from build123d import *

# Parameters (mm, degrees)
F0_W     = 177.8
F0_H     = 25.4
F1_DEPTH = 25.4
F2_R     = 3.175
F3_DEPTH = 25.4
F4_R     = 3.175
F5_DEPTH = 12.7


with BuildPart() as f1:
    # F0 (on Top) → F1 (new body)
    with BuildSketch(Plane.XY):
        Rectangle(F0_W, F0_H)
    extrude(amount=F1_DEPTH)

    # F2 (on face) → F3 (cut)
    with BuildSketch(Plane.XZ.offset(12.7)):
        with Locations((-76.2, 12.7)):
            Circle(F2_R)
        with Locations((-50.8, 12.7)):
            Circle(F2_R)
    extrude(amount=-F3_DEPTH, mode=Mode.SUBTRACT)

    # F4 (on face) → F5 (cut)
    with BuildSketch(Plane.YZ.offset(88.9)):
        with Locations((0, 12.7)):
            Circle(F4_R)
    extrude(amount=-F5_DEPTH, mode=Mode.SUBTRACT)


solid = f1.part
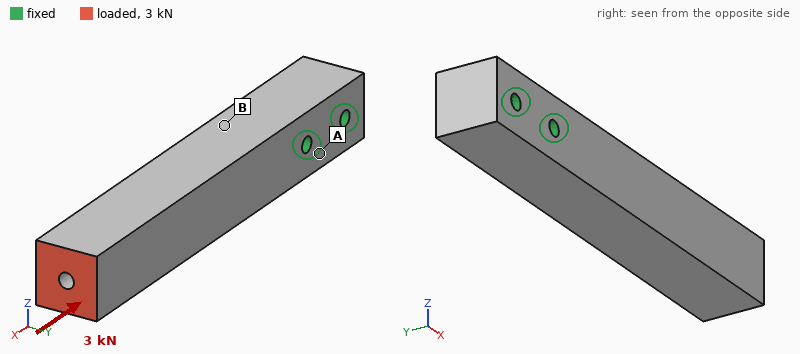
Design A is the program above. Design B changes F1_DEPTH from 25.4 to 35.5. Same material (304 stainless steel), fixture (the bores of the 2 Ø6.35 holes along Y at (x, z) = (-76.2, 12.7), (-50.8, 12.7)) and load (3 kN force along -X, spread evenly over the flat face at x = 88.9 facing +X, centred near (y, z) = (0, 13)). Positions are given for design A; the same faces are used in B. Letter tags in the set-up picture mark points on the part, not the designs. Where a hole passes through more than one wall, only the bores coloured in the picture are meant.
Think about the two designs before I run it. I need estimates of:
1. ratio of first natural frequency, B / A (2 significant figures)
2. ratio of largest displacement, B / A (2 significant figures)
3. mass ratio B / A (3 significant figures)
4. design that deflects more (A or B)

1.1
1.1
1.40
B
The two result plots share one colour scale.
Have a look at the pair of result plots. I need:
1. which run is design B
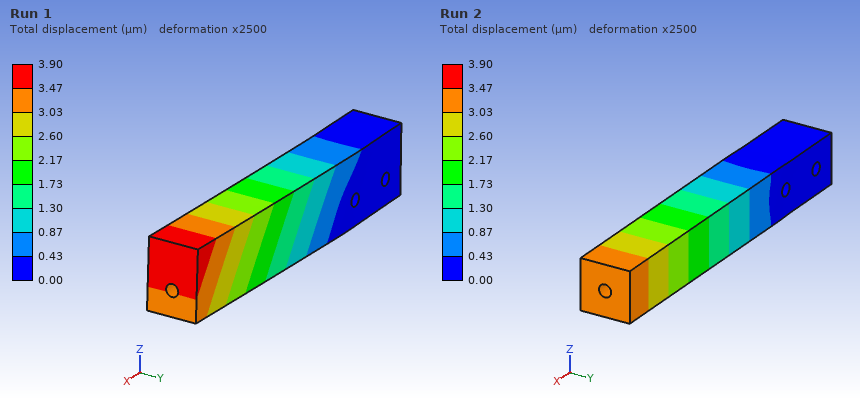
Run 1
